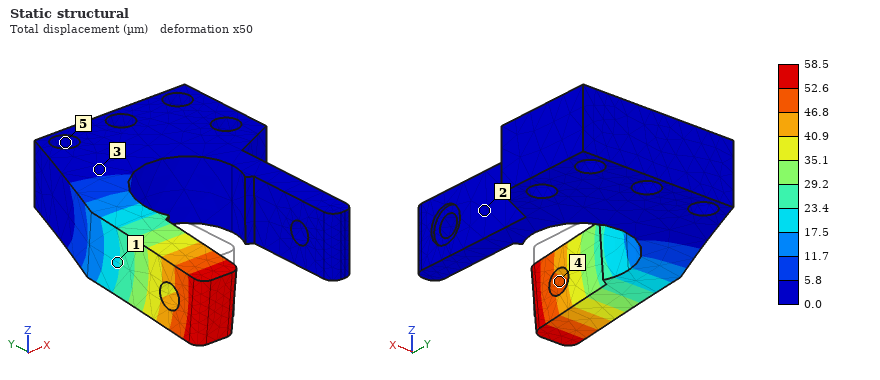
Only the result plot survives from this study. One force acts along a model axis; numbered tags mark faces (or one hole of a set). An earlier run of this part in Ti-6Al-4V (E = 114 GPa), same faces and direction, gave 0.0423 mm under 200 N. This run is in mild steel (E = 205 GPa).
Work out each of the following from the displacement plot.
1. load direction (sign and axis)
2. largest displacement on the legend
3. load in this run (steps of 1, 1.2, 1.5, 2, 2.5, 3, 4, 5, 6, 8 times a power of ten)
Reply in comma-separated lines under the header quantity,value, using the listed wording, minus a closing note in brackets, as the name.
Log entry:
quantity,value
load direction,-Z
largest displacement on the legend,58.5 µm
load in this run,500 N
